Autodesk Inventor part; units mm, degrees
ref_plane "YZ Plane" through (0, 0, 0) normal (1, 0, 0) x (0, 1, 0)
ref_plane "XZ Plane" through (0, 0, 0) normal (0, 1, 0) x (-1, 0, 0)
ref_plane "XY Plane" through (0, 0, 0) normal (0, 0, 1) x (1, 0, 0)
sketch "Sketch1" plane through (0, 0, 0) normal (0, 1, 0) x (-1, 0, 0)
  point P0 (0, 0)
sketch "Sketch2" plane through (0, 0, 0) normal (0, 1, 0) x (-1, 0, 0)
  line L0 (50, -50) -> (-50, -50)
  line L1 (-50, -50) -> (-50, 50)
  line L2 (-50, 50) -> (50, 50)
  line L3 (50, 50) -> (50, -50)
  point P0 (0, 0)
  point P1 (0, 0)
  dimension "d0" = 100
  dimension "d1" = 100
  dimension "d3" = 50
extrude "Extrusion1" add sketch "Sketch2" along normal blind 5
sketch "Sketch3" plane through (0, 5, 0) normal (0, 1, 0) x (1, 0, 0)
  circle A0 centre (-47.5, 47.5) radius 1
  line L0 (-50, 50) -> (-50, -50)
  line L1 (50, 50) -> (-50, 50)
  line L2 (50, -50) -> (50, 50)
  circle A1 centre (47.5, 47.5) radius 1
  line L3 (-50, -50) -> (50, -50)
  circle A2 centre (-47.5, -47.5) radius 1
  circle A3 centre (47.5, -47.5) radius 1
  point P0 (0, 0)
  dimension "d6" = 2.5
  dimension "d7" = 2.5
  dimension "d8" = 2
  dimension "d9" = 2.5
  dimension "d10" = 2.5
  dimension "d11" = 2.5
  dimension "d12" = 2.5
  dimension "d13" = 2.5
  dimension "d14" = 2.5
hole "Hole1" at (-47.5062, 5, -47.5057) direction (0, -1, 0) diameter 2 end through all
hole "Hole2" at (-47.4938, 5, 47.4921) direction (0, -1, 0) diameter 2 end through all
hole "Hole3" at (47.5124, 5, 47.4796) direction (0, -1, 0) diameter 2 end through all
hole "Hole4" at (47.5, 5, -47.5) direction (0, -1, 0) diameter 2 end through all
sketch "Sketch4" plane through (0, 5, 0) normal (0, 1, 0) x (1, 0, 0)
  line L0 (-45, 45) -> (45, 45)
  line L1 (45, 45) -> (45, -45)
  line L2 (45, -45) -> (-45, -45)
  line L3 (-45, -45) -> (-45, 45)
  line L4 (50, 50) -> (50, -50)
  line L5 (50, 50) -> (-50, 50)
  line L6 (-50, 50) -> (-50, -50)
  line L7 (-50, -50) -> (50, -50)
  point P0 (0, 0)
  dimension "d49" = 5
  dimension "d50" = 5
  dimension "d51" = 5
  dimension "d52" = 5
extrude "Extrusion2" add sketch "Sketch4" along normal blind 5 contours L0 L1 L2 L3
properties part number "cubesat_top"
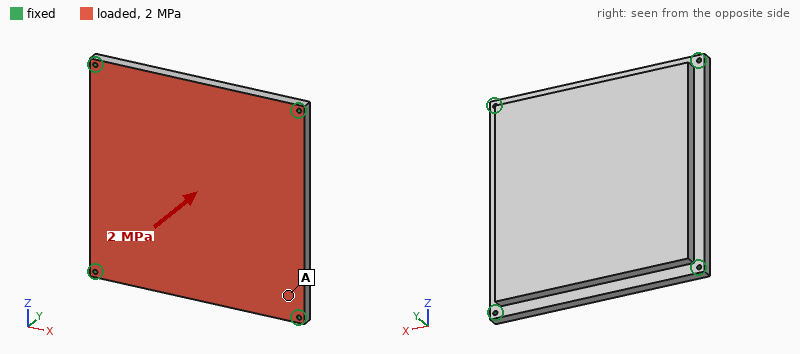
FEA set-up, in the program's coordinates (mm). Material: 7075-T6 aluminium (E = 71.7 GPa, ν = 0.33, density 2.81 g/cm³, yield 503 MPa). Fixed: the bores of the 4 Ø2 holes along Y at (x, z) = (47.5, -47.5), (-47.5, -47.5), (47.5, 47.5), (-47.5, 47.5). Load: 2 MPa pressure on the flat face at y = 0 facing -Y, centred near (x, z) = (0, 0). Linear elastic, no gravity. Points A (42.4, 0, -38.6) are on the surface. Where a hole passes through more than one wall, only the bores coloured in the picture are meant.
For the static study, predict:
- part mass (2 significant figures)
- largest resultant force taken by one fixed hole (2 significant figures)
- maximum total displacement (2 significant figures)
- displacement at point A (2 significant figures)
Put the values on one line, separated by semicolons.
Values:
250 g; 8.1 kN; 0.49 mm; 0.15 mm
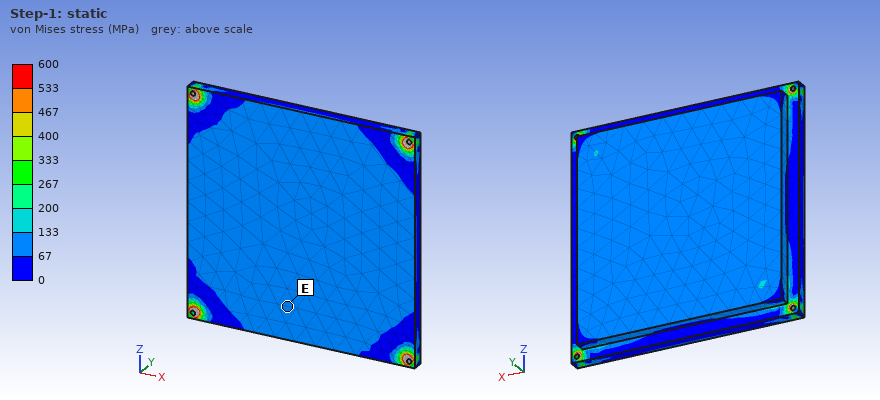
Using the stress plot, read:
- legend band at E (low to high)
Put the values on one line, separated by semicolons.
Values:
67 to 133 MPa
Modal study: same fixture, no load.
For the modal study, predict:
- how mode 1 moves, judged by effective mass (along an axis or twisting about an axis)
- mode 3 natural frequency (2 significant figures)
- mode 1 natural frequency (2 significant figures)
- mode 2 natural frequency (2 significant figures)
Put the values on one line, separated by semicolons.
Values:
along Y; 4100 Hz; 2200 Hz; 4100 Hz
